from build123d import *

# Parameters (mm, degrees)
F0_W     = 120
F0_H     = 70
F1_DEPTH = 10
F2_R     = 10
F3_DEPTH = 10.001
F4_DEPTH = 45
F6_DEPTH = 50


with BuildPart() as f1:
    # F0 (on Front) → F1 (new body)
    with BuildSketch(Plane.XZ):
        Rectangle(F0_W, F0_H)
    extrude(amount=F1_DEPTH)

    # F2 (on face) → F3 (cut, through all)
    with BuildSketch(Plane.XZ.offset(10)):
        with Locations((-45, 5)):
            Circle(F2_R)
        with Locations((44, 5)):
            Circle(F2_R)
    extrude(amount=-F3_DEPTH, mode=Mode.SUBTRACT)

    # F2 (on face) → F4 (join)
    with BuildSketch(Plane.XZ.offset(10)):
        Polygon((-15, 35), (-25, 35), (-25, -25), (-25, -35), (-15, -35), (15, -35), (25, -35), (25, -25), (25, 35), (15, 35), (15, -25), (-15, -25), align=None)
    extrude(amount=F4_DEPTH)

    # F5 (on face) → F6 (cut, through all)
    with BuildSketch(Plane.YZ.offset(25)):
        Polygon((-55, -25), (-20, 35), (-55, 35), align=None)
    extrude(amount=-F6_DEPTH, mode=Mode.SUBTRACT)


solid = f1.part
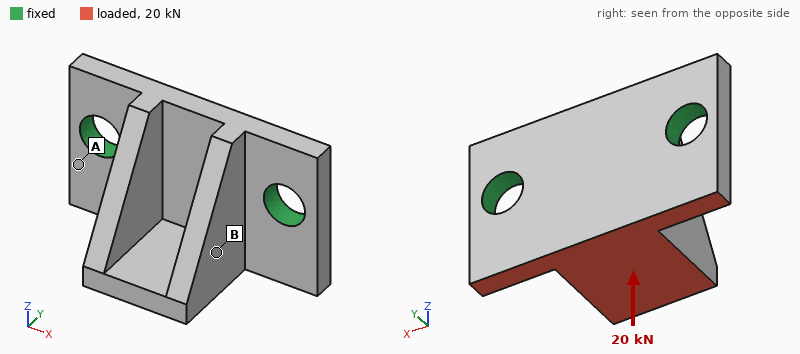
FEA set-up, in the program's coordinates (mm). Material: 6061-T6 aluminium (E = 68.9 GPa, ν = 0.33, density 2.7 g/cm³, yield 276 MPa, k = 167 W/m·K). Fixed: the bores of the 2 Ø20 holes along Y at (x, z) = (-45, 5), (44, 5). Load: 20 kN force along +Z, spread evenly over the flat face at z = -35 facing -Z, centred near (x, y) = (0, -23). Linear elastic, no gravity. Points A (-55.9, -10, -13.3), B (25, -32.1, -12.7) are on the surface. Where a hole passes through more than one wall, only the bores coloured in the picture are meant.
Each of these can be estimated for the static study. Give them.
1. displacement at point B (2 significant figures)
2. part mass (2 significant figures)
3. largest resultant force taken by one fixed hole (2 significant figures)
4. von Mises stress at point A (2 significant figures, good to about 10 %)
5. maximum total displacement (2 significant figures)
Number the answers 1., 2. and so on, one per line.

1. 0.13 mm
2. 360 g
3. 10 kN
4. 54 MPa
5. 0.29 mm
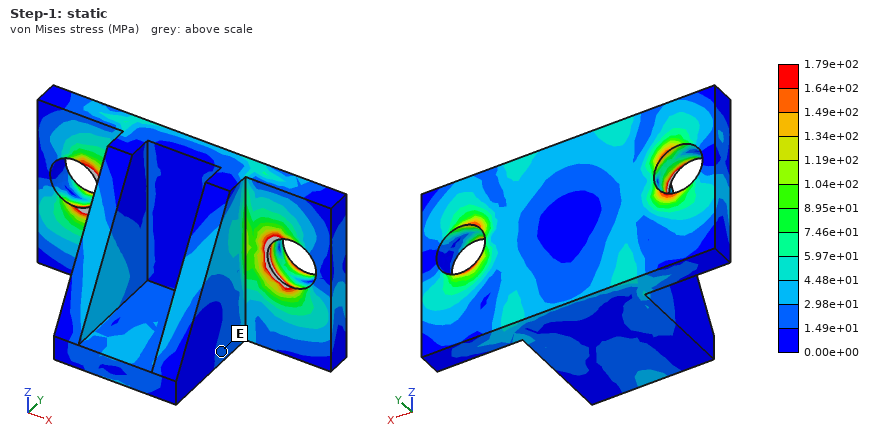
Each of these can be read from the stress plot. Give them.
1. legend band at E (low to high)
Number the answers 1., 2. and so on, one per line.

1. 1.49e+01 to 2.98e+01 MPa
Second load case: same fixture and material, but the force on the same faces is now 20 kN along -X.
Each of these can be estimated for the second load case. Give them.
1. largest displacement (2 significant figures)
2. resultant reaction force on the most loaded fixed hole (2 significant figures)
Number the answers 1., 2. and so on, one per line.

1. 0.14 mm
2. 14 kN
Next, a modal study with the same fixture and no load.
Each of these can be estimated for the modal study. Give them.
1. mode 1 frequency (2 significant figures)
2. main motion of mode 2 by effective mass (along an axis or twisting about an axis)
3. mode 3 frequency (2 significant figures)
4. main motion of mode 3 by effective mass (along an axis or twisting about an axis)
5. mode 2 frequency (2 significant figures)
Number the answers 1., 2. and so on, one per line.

1. 3000 Hz
2. along X
3. 6100 Hz
4. along Y
5. 5100 Hz
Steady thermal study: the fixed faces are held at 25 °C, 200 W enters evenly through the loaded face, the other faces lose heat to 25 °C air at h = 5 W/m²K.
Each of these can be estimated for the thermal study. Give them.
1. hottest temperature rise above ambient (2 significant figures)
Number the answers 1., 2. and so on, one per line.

1. 50 K
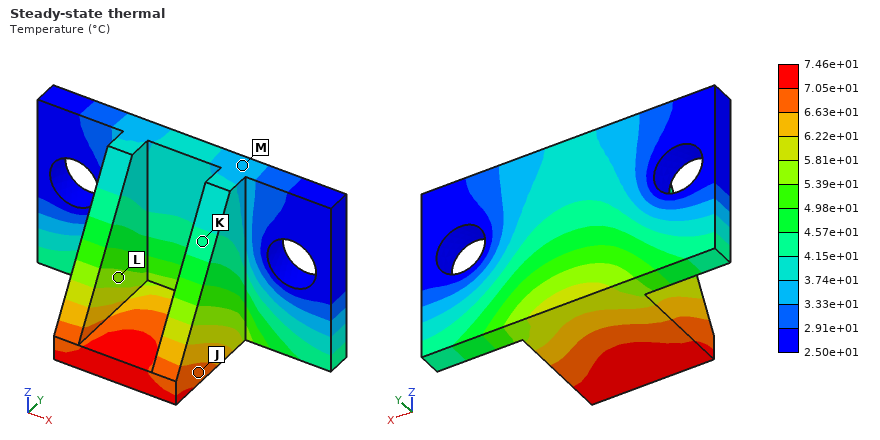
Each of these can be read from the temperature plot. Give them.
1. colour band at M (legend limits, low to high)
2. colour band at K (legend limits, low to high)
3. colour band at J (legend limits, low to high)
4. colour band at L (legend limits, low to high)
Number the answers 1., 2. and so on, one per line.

1. 3.33e+01 to 3.74e+01 °C
2. 4.15e+01 to 4.57e+01 °C
3. 6.63e+01 to 7.05e+01 °C
4. 5.39e+01 to 5.81e+01 °C
